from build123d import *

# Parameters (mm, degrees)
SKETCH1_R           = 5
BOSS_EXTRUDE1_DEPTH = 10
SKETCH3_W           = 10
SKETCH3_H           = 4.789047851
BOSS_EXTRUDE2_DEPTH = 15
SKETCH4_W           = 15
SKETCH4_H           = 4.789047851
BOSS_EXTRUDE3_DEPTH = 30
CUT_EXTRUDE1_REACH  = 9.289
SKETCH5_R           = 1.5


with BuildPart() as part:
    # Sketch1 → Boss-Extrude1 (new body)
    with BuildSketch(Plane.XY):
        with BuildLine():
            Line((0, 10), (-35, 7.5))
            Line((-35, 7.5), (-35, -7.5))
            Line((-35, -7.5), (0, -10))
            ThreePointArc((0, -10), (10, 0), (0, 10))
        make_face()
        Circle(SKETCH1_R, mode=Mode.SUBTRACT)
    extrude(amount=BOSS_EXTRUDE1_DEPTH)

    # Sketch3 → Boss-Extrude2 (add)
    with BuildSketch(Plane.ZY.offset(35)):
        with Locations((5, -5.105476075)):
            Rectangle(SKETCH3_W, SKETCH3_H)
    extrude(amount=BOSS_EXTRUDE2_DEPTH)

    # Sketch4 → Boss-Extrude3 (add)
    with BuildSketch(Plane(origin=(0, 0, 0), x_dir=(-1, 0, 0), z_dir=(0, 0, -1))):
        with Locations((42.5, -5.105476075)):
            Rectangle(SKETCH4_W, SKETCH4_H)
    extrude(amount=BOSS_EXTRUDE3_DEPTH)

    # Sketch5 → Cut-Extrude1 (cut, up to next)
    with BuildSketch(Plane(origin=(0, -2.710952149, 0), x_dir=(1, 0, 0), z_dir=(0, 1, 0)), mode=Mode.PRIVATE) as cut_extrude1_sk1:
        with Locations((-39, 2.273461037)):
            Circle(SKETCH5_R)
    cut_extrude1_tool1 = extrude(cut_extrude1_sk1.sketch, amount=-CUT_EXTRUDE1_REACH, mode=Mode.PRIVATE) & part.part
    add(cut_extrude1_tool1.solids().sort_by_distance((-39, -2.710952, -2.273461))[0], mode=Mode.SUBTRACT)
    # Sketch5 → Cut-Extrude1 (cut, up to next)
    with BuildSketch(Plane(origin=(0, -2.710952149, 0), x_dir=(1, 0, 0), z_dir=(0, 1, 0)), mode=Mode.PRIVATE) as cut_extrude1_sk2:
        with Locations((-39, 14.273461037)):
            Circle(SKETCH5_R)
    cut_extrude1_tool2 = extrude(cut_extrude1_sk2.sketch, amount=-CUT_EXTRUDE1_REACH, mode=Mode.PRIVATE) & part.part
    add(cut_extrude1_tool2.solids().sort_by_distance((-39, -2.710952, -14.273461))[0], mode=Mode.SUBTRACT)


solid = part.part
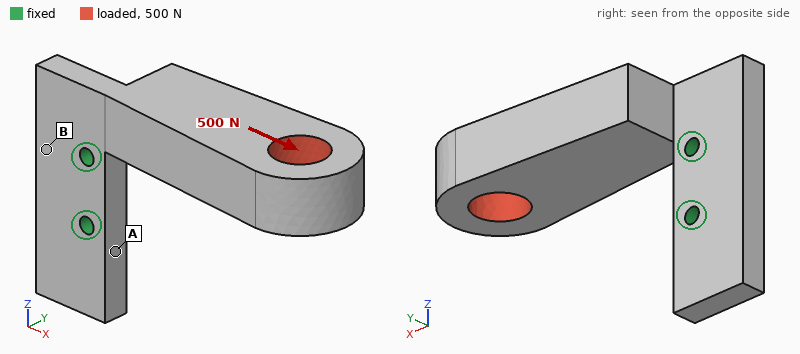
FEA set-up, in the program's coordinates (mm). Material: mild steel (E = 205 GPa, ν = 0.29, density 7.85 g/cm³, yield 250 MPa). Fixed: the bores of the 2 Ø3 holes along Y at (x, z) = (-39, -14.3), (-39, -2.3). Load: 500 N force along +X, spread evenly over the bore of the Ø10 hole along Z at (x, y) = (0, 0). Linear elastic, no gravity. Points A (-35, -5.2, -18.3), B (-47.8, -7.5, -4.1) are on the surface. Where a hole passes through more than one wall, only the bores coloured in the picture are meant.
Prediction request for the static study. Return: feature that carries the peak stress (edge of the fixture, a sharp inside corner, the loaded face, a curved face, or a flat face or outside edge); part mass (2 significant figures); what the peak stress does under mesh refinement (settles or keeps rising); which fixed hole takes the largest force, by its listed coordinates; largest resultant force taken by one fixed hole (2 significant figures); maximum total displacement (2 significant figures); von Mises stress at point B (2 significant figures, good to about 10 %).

edge of the fixture
76 g
keeps rising
(-39, -2.3)
700 N
57 µm
19 MPa
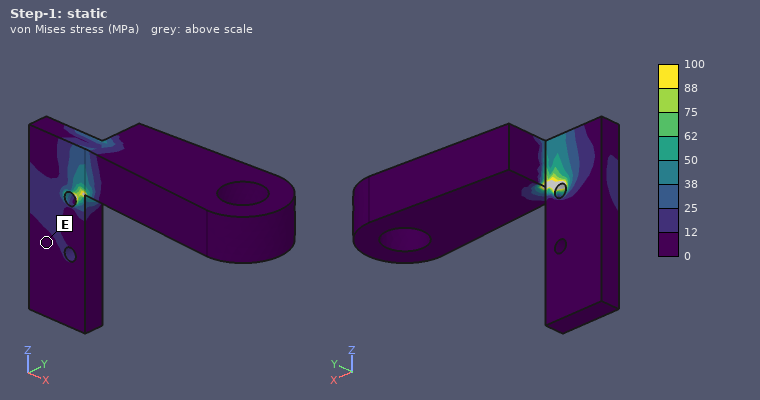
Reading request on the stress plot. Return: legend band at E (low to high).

0 to 12 MPa
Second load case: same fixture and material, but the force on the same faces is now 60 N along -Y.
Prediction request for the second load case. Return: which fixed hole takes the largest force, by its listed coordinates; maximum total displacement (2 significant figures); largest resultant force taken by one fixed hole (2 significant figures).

(-39, -2.3)
51 µm
58 N
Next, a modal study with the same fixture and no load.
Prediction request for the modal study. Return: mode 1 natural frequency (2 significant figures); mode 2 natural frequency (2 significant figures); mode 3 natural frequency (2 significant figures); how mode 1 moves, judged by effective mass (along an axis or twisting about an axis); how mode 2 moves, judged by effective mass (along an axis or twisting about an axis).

1100 Hz
1900 Hz
4900 Hz
along Y
along Z
